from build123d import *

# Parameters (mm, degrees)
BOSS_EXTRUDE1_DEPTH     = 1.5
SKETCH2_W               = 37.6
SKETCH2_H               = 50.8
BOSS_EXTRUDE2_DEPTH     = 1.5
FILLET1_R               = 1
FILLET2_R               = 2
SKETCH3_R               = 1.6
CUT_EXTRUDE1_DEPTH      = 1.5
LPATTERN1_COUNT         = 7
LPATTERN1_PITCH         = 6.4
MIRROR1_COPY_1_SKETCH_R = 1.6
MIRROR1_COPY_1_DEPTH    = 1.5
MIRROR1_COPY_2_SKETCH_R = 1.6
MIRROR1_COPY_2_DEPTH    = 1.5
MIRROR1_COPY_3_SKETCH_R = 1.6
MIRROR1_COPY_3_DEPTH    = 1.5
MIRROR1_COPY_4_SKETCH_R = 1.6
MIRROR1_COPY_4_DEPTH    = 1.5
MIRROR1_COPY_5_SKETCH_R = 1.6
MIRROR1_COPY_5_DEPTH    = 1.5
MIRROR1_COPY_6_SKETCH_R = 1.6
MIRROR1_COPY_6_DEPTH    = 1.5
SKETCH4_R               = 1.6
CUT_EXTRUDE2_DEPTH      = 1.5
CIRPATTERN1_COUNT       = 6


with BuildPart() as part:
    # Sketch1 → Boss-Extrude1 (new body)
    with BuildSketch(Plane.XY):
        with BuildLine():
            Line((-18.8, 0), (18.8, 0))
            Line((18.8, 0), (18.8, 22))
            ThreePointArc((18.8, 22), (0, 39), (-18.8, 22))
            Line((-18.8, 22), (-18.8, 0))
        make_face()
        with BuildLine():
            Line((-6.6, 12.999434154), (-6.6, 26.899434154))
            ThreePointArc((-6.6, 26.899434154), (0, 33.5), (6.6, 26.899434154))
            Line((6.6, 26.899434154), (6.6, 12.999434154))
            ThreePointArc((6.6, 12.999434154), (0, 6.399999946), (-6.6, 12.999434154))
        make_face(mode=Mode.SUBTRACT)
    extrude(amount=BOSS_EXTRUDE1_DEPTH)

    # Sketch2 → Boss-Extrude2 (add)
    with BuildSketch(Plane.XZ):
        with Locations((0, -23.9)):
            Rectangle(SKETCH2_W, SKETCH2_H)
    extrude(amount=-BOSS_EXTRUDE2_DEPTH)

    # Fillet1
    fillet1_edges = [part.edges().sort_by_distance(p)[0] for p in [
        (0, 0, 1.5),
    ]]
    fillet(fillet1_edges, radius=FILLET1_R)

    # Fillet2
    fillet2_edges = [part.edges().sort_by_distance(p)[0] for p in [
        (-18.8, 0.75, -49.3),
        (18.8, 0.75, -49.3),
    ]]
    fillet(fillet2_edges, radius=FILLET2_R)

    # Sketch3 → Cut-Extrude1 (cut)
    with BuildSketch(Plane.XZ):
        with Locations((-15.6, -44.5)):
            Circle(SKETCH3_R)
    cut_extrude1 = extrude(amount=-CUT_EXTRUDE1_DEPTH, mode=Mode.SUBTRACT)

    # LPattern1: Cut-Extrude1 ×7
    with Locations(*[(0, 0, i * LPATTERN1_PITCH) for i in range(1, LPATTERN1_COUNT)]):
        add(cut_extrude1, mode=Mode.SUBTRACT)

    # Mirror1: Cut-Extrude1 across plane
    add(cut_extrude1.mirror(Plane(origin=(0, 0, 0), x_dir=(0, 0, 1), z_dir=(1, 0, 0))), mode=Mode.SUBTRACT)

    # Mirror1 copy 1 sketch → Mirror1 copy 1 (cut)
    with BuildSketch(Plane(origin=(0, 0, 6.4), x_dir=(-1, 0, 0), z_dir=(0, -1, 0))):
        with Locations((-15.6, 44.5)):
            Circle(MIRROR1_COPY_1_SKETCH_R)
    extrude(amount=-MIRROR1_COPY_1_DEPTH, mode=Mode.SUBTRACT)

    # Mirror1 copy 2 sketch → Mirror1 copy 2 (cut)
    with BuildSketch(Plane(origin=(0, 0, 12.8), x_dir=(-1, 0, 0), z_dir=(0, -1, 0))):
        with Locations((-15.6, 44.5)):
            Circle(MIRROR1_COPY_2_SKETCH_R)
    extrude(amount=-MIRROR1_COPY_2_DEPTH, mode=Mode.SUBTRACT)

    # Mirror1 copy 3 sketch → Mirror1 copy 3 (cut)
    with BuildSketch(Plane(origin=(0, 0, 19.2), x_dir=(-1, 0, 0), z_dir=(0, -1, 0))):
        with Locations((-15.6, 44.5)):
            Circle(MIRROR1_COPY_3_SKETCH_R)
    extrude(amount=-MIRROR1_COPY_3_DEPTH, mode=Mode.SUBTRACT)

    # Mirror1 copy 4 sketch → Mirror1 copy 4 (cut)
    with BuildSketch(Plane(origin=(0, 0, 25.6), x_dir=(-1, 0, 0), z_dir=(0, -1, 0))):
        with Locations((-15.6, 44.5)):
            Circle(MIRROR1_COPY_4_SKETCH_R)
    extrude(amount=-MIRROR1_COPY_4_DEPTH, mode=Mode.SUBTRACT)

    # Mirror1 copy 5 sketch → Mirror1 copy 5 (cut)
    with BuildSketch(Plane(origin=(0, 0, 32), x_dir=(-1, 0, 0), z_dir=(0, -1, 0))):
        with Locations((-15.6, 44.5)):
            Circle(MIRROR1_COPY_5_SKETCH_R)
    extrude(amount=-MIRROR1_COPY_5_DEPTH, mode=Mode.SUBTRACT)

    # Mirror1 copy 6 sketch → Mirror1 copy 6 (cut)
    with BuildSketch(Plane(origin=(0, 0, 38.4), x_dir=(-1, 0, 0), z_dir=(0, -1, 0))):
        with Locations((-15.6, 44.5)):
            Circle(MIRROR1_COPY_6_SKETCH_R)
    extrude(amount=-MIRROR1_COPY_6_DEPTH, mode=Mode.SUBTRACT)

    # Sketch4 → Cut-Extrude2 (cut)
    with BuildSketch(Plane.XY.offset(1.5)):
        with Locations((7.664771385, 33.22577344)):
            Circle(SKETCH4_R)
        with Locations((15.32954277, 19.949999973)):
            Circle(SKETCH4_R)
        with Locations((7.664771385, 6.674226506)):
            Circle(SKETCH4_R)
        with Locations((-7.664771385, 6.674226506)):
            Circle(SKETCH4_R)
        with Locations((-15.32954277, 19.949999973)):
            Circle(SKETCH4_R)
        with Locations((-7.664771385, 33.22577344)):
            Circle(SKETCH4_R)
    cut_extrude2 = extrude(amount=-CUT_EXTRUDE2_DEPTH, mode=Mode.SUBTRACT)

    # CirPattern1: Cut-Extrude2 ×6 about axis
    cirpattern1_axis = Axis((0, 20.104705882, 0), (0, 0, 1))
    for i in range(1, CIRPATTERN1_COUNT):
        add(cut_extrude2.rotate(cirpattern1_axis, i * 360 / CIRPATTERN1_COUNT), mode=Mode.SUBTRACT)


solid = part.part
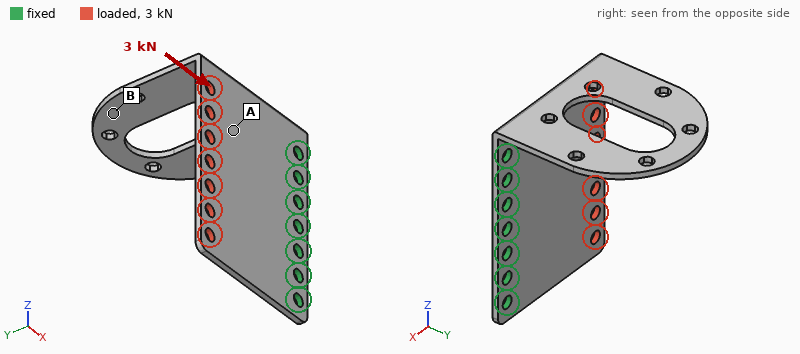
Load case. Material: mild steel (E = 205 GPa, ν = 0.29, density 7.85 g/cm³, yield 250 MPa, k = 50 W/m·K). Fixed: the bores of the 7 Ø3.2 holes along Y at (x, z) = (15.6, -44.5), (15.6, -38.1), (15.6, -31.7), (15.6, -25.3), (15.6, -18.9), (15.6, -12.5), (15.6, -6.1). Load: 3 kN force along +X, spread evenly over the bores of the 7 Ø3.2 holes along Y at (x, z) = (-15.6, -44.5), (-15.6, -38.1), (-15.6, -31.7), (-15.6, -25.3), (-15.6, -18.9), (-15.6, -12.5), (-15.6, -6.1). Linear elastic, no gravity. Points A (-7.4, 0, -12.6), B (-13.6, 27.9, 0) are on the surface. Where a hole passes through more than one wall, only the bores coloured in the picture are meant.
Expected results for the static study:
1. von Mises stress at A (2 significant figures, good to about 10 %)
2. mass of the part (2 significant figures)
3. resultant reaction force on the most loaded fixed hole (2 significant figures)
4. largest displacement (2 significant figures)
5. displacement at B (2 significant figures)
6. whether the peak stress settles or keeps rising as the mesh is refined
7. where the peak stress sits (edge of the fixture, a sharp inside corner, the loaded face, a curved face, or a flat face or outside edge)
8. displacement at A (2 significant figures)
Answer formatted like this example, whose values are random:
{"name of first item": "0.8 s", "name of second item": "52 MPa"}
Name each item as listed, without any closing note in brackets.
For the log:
{"von Mises stress at A": "44 MPa", "mass of the part": "31 g", "resultant reaction force on the most loaded fixed hole": "570 N", "largest displacement": "7.5 µm", "displacement at B": "2.1 µm", "whether the peak stress settles or keeps rising as the mesh is refined": "keeps rising", "where the peak stress sits": "edge of the fixture", "displacement at A": "4.5 µm"}
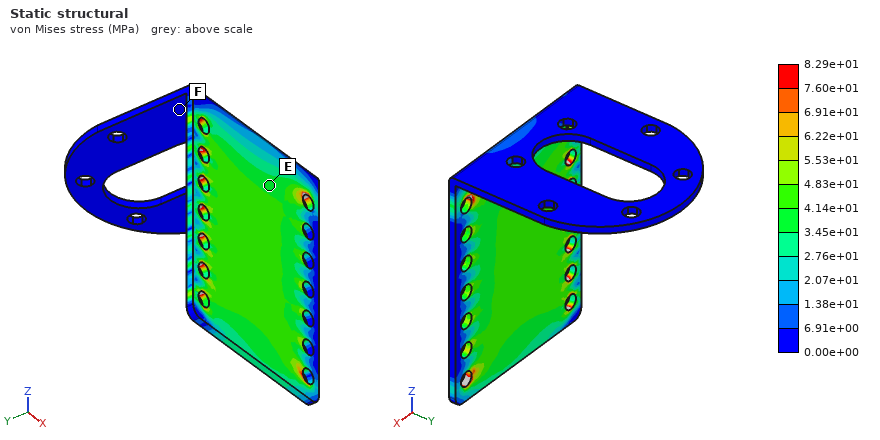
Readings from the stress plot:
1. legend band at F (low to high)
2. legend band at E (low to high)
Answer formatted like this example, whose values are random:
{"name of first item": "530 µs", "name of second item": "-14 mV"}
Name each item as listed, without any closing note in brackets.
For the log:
{"legend band at F": "0.00e+00 to 6.91e+00 MPa", "legend band at E": "3.45e+01 to 4.14e+01 MPa"}
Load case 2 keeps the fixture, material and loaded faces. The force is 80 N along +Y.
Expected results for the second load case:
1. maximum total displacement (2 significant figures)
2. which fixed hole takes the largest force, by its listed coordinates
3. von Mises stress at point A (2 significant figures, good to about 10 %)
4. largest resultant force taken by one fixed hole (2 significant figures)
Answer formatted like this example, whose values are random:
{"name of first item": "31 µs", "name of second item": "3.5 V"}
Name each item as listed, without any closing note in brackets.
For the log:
{"maximum total displacement": "0.23 mm", "which fixed hole takes the largest force, by its listed coordinates": "(15.6, -6.1)", "von Mises stress at point A": "42 MPa", "largest resultant force taken by one fixed hole": "22 N"}
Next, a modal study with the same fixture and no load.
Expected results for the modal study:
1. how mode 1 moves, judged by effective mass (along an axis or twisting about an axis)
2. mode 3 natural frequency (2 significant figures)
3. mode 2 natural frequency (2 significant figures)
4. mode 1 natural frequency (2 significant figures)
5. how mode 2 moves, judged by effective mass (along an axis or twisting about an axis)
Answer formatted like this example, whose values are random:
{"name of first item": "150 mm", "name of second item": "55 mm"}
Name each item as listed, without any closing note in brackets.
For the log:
{"how mode 1 moves, judged by effective mass": "along Z", "mode 3 natural frequency": "1600 Hz", "mode 2 natural frequency": "940 Hz", "mode 1 natural frequency": "700 Hz", "how mode 2 moves, judged by effective mass": "along Y"}
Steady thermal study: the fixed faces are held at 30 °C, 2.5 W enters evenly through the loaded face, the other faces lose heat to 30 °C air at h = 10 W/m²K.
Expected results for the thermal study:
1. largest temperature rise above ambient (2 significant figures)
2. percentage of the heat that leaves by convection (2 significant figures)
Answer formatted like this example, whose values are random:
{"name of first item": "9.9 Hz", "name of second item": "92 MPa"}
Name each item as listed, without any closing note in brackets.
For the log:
{"largest temperature rise above ambient": "20 K", "percentage of the heat that leaves by convection": "17 %"}
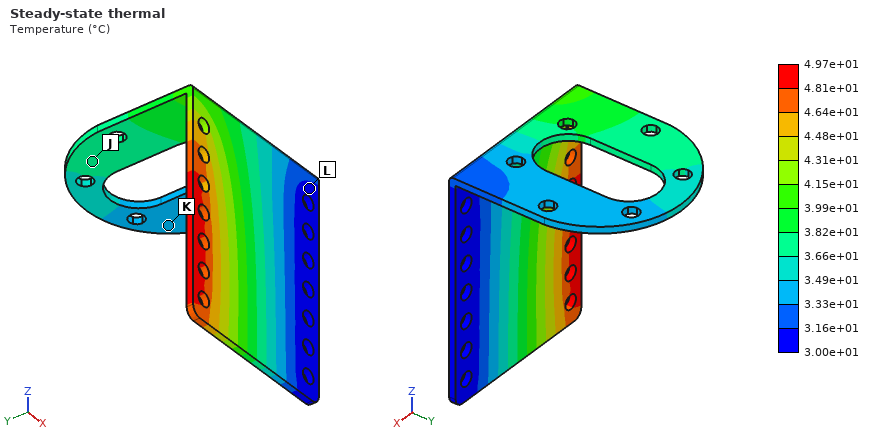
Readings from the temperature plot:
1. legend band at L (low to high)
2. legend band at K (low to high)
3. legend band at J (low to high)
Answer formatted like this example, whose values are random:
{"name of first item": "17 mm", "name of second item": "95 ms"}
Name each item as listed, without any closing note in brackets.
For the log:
{"legend band at L": "3.00e+01 to 3.16e+01 °C", "legend band at K": "3.33e+01 to 3.49e+01 °C", "legend band at J": "3.66e+01 to 3.82e+01 °C"}
